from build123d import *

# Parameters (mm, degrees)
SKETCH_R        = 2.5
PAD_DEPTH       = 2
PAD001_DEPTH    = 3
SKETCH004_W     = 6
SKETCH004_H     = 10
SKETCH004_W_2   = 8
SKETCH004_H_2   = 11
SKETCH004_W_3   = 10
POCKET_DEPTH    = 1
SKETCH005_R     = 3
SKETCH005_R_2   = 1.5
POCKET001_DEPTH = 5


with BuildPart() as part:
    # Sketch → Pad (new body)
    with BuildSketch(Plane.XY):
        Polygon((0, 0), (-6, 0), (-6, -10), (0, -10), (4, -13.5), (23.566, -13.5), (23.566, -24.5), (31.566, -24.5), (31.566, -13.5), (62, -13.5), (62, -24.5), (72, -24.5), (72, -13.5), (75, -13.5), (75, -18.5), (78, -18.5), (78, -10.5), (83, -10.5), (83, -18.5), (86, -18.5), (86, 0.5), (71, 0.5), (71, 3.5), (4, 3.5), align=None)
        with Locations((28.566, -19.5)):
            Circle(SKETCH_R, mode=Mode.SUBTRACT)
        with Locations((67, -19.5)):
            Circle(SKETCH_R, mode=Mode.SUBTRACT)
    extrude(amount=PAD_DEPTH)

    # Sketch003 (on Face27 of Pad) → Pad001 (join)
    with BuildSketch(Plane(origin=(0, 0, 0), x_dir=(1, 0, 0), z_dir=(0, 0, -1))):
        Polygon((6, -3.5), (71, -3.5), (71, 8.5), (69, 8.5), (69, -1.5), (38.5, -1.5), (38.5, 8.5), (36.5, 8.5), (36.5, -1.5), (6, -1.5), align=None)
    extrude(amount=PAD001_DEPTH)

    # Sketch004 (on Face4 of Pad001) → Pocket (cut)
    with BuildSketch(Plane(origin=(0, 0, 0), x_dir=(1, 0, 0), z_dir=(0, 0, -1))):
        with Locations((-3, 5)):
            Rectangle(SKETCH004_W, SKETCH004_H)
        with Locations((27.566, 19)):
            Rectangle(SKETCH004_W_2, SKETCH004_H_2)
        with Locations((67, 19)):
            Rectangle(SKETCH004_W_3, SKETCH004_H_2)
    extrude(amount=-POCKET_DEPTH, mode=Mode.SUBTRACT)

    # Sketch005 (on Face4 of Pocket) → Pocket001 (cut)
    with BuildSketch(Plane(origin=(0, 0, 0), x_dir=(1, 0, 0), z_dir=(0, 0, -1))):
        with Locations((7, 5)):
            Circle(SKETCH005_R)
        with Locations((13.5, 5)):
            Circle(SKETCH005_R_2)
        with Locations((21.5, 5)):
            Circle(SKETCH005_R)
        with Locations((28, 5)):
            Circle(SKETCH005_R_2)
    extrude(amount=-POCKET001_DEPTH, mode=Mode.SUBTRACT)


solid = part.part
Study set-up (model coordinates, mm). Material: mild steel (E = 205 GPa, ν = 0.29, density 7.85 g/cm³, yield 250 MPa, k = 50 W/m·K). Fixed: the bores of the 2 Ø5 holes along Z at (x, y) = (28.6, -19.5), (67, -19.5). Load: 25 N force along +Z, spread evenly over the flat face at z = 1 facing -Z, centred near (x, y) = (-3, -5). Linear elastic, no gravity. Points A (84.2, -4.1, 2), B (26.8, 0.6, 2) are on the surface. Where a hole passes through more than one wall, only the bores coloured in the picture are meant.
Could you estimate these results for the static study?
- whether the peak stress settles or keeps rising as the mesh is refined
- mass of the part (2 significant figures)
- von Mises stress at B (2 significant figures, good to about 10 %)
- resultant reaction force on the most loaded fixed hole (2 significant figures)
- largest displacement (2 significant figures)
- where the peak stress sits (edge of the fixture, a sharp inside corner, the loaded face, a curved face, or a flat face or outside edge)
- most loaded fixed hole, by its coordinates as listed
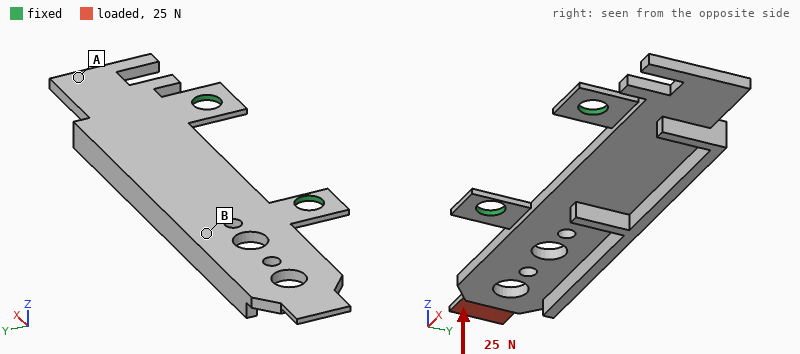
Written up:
keeps rising
27 g
34 MPa
42 N
0.22 mm
edge of the fixture
(28.6, -19.5)
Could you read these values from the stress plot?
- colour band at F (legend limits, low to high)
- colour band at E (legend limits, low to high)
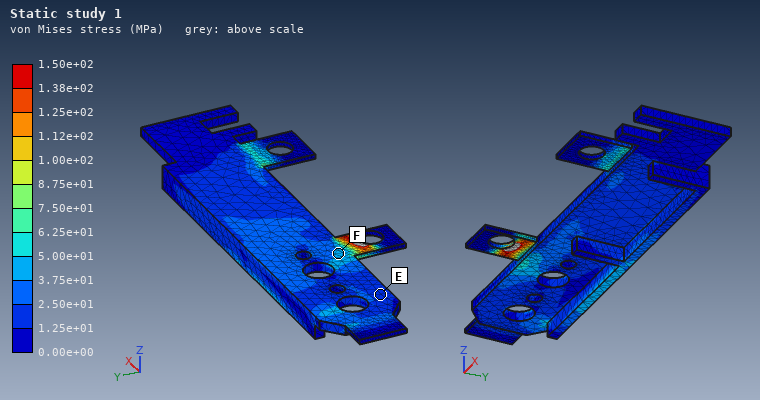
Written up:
3.75e+01 to 5.00e+01 MPa
1.25e+01 to 2.50e+01 MPa
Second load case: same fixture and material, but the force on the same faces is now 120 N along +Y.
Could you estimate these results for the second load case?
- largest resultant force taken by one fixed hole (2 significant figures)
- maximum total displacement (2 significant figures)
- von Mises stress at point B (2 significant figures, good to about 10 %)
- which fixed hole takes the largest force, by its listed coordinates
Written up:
220 N
60 µm
26 MPa
(28.6, -19.5)
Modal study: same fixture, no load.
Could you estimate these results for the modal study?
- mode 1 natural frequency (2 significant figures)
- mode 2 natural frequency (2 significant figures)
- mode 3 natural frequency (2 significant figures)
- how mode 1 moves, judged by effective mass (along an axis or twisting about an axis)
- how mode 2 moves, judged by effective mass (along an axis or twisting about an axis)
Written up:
660 Hz
1400 Hz
2700 Hz
along Z
twisting about Y
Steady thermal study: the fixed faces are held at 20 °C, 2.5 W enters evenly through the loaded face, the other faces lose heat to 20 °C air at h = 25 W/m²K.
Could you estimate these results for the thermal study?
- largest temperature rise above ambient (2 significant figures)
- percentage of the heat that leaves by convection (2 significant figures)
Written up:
67 K
54 %
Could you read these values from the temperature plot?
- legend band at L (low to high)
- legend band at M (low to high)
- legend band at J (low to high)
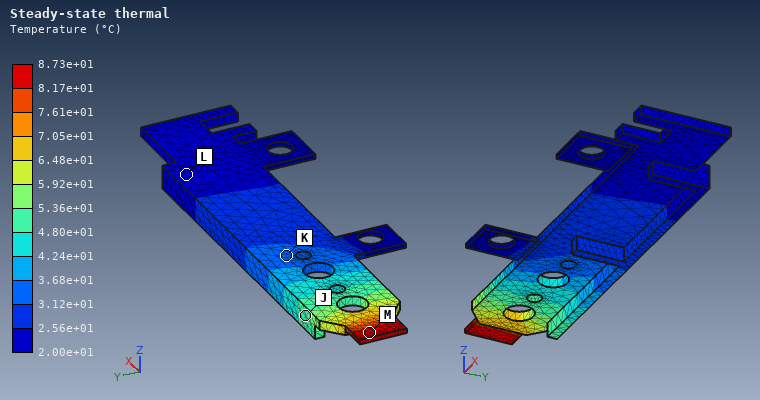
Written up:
2.00e+01 to 2.56e+01 °C
8.17e+01 to 8.73e+01 °C
4.80e+01 to 5.36e+01 °C
